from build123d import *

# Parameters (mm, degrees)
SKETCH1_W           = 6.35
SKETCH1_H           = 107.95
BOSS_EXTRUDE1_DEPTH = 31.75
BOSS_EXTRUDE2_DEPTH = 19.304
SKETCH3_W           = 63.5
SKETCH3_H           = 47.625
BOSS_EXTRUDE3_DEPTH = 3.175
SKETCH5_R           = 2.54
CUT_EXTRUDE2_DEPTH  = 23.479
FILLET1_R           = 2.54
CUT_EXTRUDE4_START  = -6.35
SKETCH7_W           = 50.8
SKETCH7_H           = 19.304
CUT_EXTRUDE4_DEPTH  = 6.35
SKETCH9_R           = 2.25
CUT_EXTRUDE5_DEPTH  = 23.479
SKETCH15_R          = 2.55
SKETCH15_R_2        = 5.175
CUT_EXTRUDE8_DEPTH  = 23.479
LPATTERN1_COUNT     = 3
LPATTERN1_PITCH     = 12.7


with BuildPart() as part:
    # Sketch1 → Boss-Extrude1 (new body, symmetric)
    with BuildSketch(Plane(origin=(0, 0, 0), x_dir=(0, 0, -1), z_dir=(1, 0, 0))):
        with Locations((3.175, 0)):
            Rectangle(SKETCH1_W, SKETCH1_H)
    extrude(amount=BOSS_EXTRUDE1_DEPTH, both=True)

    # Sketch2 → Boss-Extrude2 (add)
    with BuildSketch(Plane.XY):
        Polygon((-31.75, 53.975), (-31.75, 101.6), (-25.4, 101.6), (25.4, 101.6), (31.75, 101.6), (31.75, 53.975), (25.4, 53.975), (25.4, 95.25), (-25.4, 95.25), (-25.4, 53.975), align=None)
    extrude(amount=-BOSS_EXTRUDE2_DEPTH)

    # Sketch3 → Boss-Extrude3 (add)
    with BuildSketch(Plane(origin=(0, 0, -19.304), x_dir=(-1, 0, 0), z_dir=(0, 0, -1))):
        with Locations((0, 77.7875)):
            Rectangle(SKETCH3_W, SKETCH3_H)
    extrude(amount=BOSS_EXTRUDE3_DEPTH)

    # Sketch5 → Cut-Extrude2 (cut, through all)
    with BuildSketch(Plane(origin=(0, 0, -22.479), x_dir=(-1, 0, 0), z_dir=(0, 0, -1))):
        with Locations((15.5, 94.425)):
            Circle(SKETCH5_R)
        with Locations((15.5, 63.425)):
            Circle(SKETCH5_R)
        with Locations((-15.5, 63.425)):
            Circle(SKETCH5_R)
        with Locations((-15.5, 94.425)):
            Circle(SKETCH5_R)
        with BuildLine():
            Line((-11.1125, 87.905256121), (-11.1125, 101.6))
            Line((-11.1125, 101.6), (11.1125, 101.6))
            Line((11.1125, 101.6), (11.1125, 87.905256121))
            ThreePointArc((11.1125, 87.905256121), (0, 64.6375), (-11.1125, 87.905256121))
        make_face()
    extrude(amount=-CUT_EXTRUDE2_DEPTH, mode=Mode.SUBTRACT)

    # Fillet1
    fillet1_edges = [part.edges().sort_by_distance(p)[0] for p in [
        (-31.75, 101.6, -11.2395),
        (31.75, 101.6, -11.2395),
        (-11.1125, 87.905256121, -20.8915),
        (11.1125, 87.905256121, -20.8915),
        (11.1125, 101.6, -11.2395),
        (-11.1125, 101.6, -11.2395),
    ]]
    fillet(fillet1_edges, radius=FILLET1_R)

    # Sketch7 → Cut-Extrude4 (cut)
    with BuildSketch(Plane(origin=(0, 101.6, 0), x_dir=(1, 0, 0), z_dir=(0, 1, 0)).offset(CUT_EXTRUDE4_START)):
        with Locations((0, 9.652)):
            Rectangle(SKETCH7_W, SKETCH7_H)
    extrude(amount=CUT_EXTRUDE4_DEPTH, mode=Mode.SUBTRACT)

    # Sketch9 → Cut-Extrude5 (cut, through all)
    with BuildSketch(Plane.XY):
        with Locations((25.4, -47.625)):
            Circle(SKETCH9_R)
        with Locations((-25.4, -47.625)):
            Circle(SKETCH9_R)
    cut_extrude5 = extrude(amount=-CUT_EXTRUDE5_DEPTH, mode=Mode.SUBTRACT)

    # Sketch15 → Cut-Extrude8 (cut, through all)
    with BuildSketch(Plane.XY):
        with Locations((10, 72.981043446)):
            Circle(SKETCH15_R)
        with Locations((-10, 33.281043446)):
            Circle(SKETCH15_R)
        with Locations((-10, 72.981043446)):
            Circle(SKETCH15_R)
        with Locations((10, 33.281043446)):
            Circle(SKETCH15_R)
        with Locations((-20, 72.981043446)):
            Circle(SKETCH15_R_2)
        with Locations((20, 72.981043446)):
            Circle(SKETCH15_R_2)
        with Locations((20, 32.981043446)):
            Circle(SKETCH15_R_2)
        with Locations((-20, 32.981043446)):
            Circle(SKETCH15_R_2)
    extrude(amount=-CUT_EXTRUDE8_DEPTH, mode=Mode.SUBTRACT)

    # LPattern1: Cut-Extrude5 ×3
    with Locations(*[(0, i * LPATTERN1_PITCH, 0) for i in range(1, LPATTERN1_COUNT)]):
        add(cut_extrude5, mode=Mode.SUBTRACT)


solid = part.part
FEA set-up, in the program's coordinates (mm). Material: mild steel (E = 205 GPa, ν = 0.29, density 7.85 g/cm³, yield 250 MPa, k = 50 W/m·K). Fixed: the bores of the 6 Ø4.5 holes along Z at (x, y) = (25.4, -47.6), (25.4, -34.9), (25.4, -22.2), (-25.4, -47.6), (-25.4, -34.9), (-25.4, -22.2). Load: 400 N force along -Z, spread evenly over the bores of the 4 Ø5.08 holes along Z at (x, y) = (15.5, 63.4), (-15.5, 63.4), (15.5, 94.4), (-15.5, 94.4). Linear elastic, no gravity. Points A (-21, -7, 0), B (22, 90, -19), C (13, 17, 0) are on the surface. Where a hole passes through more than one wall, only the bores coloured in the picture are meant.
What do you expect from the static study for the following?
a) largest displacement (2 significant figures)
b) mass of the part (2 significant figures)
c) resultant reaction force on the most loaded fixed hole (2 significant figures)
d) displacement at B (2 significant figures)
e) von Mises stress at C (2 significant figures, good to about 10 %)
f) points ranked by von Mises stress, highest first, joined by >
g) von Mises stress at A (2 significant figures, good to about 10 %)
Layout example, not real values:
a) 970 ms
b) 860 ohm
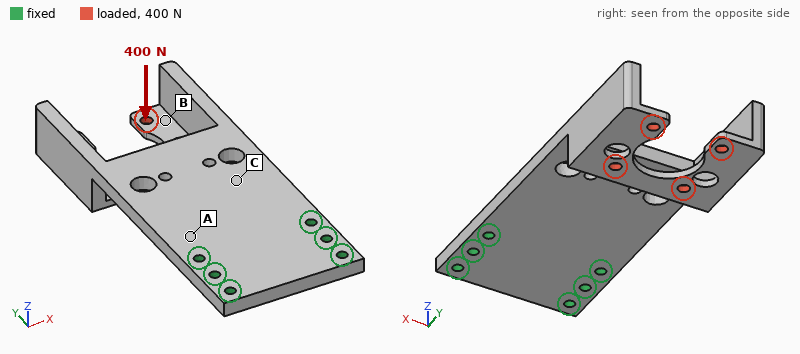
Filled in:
a) 0.84 mm
b) 470 g
c) 750 N
d) 0.72 mm
e) 56 MPa
f) A > C > B
g) 80 MPa
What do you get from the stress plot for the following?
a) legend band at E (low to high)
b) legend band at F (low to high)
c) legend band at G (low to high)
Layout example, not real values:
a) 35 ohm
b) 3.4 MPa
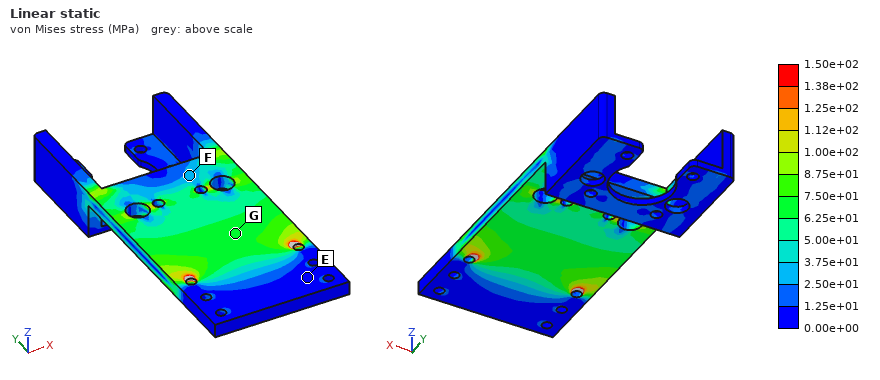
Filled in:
a) 0.00e+00 to 1.25e+01 MPa
b) 2.50e+01 to 3.75e+01 MPa
c) 6.25e+01 to 7.50e+01 MPa
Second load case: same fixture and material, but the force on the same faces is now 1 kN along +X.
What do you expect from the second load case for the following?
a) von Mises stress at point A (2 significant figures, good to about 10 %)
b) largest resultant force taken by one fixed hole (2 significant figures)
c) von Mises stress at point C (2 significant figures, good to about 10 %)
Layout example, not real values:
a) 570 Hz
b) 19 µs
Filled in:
a) 34 MPa
b) 1.8 kN
c) 28 MPa
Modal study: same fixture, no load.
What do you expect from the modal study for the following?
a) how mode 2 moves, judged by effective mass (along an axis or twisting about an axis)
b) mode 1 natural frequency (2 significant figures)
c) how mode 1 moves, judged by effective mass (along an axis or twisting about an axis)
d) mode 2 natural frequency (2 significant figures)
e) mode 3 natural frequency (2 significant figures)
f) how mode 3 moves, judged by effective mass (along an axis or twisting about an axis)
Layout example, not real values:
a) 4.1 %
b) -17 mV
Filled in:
a) twisting about Y
b) 330 Hz
c) along Z
d) 780 Hz
e) 1400 Hz
f) along X
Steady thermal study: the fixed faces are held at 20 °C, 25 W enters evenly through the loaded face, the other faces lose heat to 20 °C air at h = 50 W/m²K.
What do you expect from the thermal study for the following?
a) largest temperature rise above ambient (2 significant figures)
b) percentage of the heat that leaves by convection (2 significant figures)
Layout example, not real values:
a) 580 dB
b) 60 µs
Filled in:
a) 70 K
b) 91 %
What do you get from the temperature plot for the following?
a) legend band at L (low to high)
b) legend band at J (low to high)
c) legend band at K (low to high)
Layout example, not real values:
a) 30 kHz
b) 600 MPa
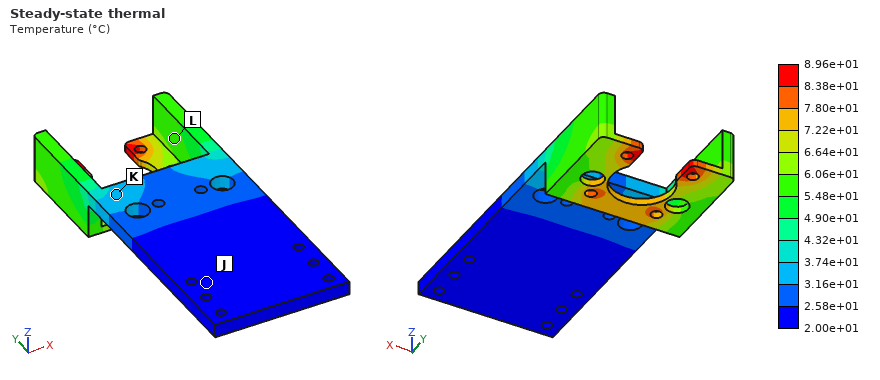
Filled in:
a) 5.48e+01 to 6.06e+01 °C
b) 2.00e+01 to 2.58e+01 °C
c) 3.16e+01 to 3.74e+01 °C
